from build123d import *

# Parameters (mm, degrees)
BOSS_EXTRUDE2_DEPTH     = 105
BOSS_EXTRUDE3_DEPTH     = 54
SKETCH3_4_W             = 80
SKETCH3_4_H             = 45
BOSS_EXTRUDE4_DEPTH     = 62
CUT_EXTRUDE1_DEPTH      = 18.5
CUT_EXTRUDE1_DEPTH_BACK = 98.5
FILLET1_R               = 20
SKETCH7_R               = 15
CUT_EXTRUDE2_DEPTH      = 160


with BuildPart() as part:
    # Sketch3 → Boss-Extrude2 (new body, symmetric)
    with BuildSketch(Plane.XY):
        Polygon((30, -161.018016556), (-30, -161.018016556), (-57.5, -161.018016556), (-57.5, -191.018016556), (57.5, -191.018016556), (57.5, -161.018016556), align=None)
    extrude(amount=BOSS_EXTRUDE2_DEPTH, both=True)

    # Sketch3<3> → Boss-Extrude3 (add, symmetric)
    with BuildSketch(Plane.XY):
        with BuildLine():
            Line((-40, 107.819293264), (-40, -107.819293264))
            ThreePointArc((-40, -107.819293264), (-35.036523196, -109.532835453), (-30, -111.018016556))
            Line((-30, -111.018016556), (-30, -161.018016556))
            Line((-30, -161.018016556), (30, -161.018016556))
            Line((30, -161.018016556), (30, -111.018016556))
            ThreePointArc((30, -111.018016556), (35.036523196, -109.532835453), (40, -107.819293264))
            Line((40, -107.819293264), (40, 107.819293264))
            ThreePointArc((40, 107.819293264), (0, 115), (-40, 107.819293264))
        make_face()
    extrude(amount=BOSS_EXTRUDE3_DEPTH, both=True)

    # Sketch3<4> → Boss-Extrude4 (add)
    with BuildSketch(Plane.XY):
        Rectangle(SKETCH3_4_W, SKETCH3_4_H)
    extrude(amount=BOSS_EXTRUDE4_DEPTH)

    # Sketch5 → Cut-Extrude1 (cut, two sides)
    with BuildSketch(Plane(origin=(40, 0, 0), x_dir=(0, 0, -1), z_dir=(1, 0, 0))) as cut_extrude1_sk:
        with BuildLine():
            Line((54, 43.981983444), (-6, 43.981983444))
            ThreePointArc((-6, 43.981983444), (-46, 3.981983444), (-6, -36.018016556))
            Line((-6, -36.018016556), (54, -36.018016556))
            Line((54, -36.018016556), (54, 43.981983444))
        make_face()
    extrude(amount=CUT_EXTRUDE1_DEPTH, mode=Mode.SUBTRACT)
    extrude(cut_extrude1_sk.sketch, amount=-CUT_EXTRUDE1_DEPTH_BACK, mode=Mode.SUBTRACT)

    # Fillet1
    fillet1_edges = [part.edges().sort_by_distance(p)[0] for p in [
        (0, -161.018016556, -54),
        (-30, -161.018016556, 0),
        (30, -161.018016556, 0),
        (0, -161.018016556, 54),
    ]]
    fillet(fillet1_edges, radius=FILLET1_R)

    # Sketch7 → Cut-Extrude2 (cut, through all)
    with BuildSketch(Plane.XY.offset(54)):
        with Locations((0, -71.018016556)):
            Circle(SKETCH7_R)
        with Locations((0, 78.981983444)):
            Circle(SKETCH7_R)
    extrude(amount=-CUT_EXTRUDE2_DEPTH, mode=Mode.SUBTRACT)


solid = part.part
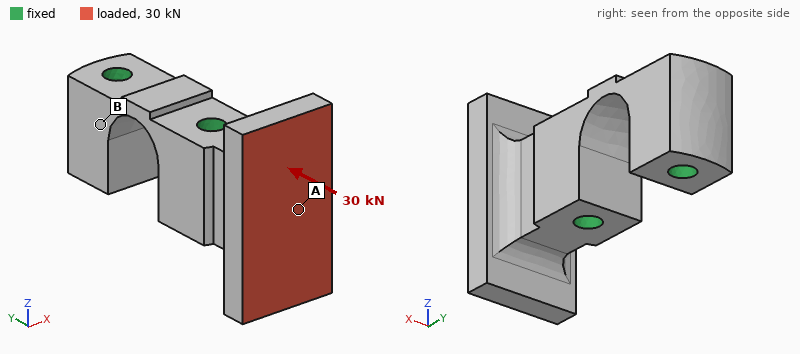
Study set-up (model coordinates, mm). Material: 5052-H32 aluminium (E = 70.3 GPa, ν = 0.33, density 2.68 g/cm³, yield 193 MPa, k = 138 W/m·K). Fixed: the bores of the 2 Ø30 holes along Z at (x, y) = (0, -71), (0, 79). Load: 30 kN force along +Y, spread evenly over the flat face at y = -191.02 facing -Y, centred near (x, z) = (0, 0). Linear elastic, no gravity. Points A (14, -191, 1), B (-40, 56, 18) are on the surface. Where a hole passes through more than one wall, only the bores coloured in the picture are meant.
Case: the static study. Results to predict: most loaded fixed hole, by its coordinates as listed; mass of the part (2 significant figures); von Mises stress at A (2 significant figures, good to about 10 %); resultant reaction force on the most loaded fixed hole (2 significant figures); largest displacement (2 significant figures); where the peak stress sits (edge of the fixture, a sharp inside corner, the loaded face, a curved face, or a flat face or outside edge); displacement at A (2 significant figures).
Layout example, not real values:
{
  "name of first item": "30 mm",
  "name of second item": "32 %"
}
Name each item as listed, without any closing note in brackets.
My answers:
{
  "most loaded fixed hole, by its coordinates as listed": "(0, -71)",
  "mass of the part": "6.2 kg",
  "von Mises stress at A": "5.9 MPa",
  "resultant reaction force on the most loaded fixed hole": "30 kN",
  "largest displacement": "25 µm",
  "where the peak stress sits": "a curved face",
  "displacement at A": "4.2 µm"
}
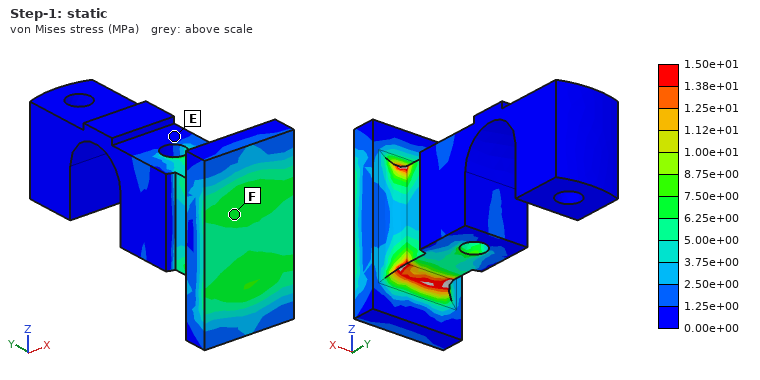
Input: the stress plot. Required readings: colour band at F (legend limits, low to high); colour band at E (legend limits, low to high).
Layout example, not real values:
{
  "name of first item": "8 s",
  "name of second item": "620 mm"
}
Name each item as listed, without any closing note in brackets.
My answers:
{
  "colour band at F": "6.25e+00 to 7.50e+00 MPa",
  "colour band at E": "0.00e+00 to 1.25e+00 MPa"
}
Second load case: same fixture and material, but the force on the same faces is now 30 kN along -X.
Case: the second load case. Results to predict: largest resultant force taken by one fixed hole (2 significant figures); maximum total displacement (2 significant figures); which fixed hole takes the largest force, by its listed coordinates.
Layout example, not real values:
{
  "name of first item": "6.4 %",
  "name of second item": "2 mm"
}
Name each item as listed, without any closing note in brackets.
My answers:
{
  "largest resultant force taken by one fixed hole": "33 kN",
  "maximum total displacement": "0.16 mm",
  "which fixed hole takes the largest force, by its listed coordinates": "(0, -71)"
}
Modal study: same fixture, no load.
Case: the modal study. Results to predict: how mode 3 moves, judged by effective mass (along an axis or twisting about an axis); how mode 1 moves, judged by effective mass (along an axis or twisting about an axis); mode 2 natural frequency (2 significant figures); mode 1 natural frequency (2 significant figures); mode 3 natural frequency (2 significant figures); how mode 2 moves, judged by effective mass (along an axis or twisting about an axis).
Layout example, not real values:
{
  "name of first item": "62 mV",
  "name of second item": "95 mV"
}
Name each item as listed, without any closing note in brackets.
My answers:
{
  "how mode 3 moves, judged by effective mass": "along Z",
  "how mode 1 moves, judged by effective mass": "along X",
  "mode 2 natural frequency": "2300 Hz",
  "mode 1 natural frequency": "1800 Hz",
  "mode 3 natural frequency": "2500 Hz",
  "how mode 2 moves, judged by effective mass": "twisting about Y"
}
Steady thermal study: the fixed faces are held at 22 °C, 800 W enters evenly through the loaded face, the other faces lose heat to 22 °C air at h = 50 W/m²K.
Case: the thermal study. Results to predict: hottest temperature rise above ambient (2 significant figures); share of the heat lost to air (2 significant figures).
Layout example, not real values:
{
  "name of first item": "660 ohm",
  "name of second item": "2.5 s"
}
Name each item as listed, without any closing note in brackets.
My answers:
{
  "hottest temperature rise above ambient": "74 K",
  "share of the heat lost to air": "20 %"
}
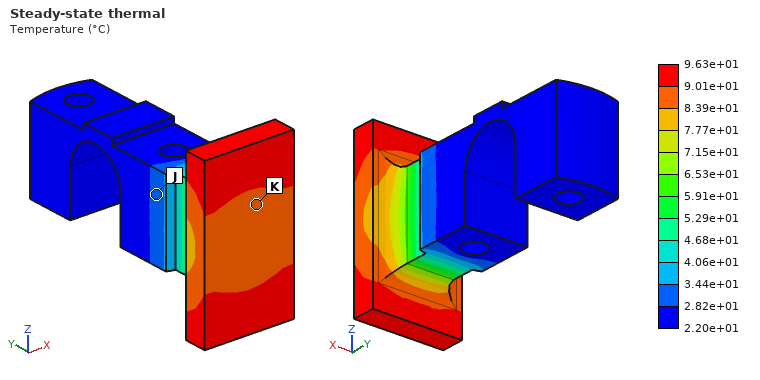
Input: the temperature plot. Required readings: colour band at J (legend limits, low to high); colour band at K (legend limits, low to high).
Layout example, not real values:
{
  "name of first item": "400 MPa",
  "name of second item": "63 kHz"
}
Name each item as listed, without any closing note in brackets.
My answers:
{
  "colour band at J": "2.82e+01 to 3.44e+01 °C",
  "colour band at K": "8.39e+01 to 9.01e+01 °C"
}
